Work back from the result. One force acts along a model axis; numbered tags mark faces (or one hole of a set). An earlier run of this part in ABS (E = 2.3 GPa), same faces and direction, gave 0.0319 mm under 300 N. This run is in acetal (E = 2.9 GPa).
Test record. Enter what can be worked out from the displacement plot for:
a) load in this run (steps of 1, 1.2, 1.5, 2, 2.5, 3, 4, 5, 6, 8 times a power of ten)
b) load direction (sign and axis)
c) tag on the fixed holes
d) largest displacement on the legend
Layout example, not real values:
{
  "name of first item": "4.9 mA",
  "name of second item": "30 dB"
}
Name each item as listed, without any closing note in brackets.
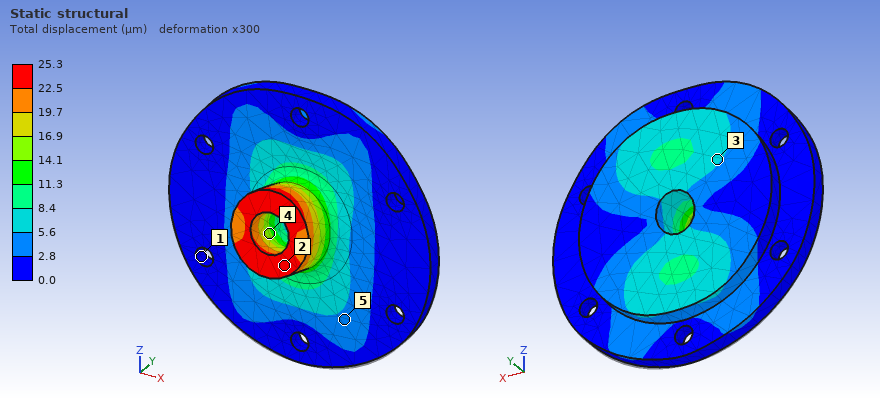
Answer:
{
  "load in this run": "300 N",
  "load direction": "+Z",
  "tag on the fixed holes": "1",
  "largest displacement on the legend": "25.3 µm"
}
